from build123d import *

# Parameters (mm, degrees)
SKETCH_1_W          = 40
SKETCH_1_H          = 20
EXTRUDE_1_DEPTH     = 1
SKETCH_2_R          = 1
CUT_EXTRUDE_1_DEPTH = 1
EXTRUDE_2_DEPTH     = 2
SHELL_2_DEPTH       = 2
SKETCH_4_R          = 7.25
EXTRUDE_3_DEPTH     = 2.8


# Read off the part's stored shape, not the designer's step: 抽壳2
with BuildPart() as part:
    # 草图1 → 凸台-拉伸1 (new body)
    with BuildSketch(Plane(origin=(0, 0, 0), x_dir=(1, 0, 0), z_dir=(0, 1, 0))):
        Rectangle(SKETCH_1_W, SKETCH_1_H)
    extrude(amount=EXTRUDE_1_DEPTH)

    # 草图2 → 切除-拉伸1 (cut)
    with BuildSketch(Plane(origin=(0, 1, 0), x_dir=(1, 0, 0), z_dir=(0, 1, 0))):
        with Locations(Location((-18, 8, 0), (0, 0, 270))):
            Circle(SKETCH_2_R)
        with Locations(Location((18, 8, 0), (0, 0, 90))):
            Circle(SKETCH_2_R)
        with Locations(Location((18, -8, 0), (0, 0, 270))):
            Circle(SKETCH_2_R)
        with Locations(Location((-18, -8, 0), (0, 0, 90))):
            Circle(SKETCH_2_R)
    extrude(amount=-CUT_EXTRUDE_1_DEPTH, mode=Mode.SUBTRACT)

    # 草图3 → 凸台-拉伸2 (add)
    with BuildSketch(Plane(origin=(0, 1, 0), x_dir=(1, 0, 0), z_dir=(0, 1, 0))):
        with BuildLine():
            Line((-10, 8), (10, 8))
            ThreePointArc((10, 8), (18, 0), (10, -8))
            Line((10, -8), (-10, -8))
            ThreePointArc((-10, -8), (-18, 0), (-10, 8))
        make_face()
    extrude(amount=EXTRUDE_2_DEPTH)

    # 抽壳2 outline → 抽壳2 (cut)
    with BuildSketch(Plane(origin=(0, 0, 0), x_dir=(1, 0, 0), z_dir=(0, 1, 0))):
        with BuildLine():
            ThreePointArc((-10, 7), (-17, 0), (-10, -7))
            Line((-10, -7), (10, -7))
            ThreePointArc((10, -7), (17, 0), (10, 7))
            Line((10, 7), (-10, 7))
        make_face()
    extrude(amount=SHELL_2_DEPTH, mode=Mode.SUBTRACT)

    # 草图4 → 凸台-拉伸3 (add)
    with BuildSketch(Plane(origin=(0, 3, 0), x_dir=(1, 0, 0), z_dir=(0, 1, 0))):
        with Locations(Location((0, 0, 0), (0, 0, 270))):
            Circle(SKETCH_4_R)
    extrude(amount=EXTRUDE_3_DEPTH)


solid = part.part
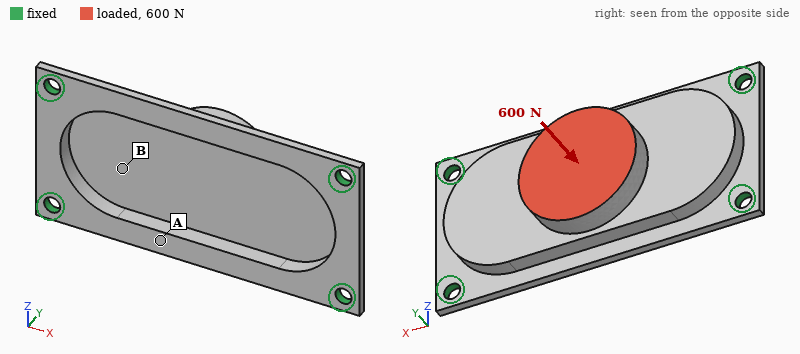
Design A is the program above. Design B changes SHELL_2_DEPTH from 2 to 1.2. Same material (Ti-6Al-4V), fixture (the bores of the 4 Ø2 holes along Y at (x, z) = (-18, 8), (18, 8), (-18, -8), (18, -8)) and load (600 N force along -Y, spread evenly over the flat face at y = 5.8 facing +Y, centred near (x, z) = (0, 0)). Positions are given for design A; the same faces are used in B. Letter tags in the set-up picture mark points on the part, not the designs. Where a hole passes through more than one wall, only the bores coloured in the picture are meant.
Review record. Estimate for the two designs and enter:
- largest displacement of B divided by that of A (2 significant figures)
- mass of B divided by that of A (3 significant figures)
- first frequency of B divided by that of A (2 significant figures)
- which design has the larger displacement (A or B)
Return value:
0.73
1.24
1.1
A
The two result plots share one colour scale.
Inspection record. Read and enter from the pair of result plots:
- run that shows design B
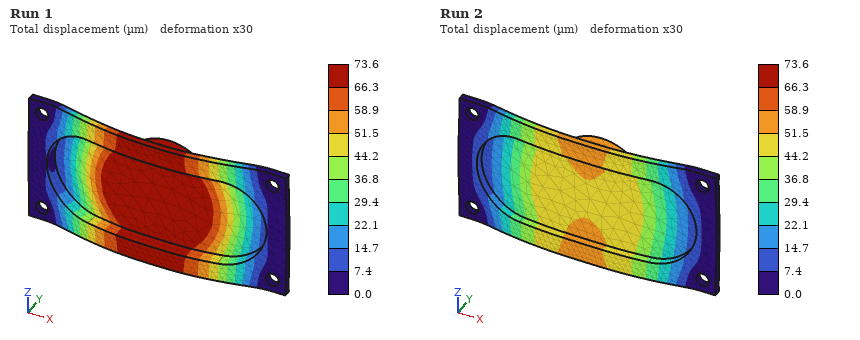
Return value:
Run 2
